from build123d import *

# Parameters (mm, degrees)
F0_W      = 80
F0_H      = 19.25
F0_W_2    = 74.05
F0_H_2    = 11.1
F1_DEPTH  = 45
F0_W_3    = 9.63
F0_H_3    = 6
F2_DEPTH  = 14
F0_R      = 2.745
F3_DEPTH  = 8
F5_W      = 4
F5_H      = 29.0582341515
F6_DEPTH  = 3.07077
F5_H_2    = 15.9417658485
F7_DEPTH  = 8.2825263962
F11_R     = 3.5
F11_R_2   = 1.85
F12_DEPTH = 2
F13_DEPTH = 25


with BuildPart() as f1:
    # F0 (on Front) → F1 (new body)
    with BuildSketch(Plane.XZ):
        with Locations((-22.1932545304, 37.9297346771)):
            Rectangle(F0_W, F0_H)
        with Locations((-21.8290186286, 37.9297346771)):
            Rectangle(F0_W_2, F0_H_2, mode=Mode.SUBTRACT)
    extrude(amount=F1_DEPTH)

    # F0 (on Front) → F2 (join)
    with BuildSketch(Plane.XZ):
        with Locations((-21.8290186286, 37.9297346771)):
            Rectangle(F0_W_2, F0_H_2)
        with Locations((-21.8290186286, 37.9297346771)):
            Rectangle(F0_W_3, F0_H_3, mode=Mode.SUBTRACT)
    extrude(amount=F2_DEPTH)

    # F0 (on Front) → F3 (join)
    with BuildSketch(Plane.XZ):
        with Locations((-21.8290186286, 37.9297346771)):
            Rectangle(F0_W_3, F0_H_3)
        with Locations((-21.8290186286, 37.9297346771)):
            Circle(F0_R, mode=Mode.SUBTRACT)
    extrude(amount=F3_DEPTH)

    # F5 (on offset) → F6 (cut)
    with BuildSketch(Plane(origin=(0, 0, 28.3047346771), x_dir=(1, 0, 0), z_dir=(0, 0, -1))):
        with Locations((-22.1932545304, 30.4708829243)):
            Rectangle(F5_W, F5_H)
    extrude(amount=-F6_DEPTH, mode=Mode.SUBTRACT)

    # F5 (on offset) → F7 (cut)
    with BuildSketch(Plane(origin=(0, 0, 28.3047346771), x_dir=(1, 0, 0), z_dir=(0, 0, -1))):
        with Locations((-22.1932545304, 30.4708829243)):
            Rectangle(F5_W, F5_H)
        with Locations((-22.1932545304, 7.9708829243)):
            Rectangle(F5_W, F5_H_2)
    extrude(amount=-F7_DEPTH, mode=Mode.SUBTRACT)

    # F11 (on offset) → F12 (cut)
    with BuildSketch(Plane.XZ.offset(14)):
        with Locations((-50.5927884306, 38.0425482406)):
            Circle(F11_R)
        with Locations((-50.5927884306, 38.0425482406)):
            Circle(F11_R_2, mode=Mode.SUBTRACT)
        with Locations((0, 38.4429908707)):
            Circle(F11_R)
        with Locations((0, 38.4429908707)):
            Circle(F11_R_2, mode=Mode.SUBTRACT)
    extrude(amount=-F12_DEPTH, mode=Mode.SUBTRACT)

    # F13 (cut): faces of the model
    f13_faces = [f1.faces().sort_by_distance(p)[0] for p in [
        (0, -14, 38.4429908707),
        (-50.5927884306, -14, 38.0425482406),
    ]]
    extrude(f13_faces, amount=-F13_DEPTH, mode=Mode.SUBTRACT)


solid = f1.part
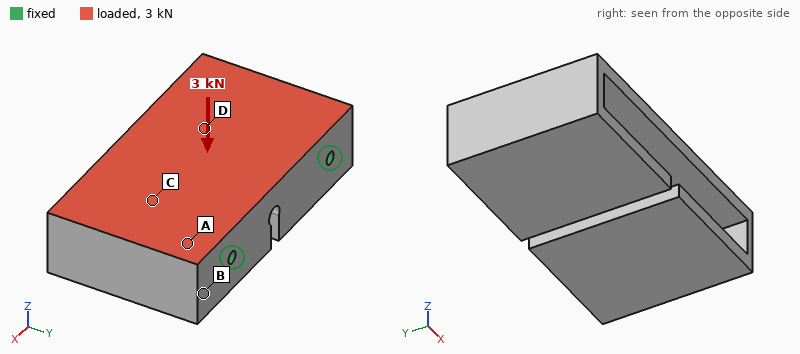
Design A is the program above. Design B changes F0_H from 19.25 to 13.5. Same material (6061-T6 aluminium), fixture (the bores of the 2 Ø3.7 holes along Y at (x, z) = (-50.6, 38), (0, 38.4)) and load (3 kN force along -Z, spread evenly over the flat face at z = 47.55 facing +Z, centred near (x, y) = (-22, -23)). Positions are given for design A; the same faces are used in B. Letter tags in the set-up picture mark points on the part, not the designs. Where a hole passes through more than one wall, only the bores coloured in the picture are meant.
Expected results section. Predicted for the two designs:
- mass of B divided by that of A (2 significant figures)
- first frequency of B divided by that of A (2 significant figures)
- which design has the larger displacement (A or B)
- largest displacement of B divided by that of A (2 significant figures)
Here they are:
0.52
0.47
B
19
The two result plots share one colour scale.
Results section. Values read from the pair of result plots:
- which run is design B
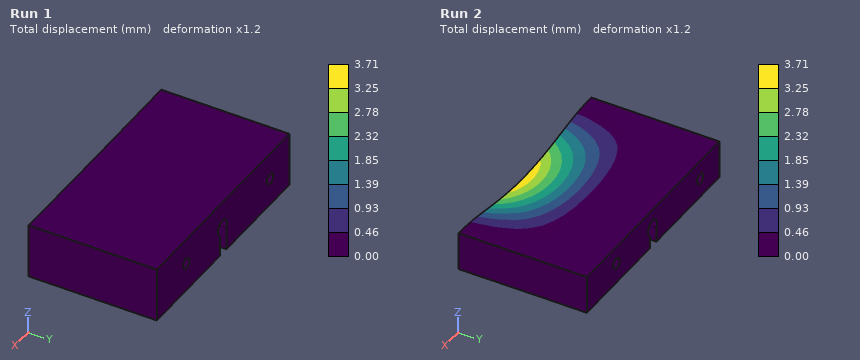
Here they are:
Run 2
